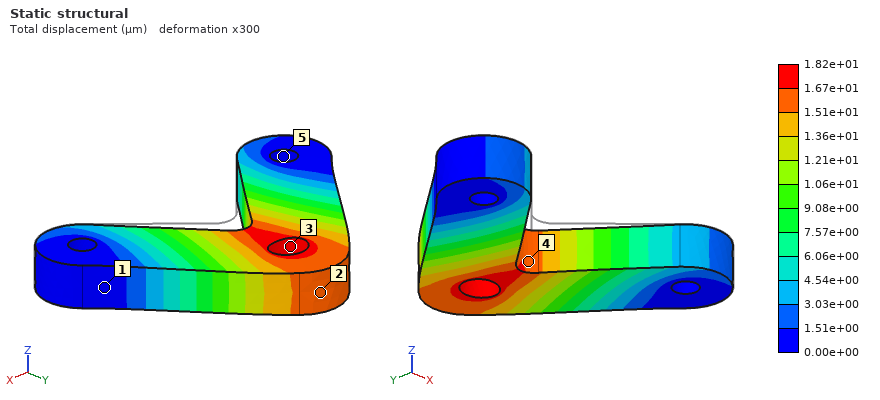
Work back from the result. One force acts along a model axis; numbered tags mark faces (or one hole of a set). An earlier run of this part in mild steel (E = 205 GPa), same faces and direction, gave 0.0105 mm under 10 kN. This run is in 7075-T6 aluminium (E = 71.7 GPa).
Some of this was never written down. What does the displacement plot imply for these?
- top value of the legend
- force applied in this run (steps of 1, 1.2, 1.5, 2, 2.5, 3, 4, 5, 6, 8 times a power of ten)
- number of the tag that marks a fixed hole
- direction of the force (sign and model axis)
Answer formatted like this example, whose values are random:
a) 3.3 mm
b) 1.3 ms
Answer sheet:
a) 1.82e+01 µm
b) 6 kN
c) 5
d) +Y
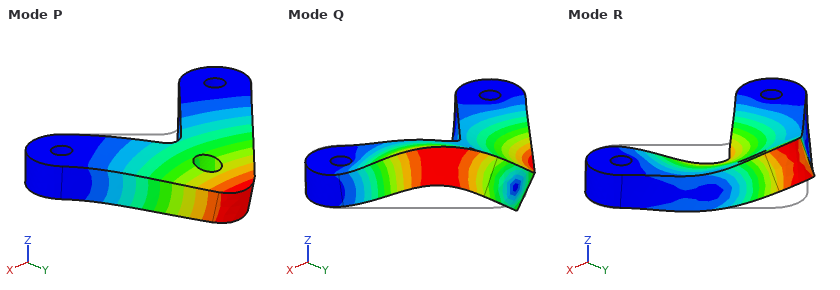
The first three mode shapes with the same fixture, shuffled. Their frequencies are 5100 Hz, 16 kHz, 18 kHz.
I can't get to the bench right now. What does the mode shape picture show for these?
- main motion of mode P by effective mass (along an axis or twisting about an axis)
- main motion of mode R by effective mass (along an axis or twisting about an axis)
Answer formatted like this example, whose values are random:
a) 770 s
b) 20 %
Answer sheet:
a) along Z
b) along Z
